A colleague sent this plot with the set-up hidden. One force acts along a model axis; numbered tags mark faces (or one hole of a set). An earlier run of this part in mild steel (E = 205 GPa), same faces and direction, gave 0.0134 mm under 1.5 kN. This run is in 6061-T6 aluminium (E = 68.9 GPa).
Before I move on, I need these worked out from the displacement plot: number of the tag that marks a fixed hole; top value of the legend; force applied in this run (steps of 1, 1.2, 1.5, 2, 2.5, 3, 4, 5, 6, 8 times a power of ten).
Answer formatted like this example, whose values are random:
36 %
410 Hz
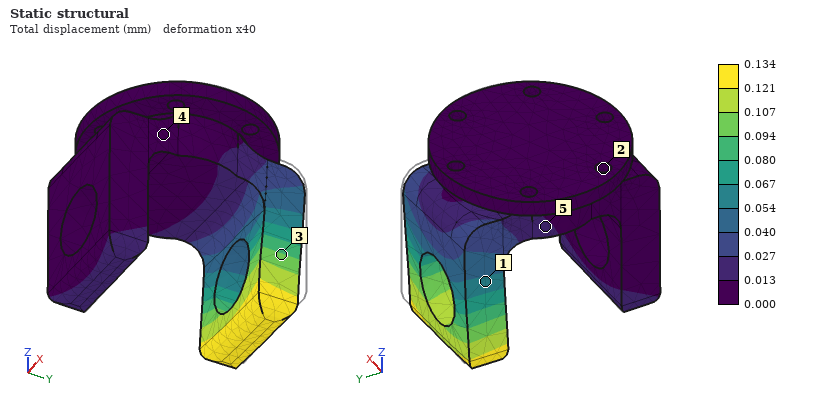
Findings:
2
0.134 mm
5 kN
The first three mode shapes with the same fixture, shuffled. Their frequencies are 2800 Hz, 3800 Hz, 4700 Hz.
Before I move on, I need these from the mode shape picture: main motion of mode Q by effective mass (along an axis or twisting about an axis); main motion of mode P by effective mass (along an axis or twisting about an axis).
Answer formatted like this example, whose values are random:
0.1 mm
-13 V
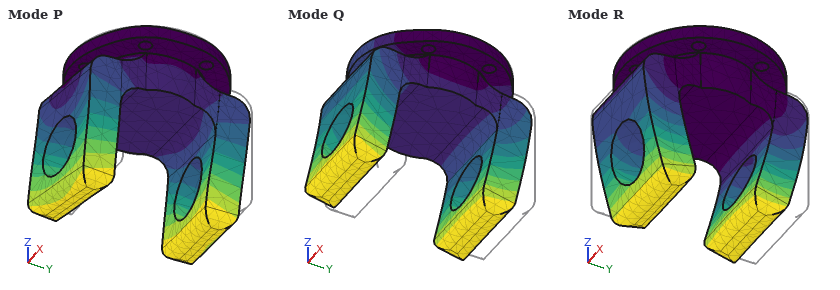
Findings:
along Y
along X
